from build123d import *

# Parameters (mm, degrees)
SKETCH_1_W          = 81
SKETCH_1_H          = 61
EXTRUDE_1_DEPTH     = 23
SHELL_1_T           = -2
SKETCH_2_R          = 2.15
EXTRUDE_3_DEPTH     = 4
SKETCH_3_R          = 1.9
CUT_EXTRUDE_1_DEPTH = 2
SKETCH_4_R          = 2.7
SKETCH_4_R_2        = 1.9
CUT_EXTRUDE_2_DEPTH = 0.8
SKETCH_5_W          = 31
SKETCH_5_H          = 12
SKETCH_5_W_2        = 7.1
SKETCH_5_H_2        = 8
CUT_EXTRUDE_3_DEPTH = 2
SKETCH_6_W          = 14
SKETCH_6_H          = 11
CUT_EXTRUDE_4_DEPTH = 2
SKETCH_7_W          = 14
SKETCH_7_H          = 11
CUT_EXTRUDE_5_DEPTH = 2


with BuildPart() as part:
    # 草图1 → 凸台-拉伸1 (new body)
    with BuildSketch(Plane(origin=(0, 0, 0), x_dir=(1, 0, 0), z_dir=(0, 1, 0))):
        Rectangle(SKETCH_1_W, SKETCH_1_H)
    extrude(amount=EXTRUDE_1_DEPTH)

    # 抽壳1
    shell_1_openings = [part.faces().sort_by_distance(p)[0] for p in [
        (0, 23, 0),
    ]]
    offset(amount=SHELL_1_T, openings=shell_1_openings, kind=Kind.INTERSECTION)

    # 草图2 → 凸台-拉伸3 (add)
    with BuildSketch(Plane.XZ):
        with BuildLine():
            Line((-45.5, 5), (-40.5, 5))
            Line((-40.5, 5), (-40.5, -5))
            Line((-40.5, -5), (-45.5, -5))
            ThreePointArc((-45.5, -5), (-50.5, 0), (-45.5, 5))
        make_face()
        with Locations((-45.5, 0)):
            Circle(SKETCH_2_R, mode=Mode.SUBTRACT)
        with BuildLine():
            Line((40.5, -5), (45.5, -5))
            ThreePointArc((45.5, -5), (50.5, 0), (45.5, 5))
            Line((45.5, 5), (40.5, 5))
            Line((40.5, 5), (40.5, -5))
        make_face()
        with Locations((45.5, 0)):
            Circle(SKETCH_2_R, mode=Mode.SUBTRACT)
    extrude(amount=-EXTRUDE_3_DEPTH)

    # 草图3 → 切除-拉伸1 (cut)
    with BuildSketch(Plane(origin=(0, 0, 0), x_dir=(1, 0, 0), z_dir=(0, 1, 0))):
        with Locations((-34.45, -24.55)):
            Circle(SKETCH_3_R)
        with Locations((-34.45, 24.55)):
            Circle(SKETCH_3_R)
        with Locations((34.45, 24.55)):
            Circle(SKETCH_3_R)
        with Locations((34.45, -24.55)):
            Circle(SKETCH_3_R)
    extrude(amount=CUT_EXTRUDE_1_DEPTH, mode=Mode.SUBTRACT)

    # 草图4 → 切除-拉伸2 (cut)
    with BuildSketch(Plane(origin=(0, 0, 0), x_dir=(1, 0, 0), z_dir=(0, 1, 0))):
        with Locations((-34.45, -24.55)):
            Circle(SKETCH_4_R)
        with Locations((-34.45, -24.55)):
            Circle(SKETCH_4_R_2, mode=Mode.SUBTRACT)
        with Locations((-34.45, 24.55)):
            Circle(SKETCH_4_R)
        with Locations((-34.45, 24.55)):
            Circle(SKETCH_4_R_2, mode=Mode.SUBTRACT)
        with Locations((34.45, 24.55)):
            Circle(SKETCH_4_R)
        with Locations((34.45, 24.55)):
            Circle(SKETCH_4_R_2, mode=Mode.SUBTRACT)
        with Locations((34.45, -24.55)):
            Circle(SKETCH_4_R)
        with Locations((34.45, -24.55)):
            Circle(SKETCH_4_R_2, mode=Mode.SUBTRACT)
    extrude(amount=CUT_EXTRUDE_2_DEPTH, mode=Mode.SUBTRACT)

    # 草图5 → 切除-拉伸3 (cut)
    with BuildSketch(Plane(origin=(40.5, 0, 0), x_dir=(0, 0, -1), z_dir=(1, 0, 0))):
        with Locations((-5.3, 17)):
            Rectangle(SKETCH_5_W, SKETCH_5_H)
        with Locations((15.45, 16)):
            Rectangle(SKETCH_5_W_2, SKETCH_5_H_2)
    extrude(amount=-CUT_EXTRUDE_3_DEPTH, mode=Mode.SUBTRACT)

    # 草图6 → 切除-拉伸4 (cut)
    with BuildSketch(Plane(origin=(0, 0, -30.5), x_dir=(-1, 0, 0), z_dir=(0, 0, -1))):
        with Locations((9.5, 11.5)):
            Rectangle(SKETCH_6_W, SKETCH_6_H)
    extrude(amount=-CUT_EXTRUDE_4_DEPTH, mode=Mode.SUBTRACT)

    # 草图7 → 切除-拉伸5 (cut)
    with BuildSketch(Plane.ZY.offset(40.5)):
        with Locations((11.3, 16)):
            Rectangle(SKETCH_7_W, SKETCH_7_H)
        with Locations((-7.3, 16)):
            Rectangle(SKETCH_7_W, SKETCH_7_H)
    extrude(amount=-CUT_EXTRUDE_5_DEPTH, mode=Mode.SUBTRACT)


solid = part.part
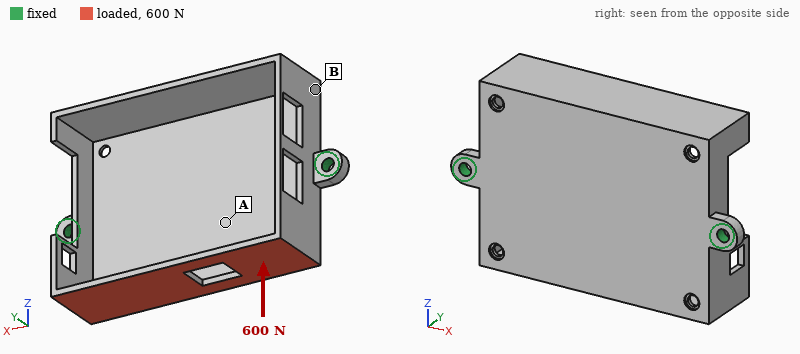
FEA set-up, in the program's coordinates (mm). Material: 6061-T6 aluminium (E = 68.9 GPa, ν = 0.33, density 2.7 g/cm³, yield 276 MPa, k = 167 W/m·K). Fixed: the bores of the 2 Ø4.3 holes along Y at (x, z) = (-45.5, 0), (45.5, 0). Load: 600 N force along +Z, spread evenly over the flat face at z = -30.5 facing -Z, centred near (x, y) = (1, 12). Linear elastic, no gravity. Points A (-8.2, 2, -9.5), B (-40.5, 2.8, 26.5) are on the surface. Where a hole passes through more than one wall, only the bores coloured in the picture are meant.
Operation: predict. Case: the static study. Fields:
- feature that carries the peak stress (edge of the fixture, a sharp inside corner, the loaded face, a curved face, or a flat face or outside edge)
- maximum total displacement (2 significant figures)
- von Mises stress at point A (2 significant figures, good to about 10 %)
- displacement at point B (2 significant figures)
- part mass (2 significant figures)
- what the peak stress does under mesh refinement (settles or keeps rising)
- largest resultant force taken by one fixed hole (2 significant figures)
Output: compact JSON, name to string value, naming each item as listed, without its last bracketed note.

{"feature that carries the peak stress": "edge of the fixture", "maximum total displacement": "0.41 mm", "von Mises stress at point A": "17 MPa", "displacement at point B": "0.079 mm", "part mass": "54 g", "what the peak stress does under mesh refinement": "keeps rising", "largest resultant force taken by one fixed hole": "310 N"}
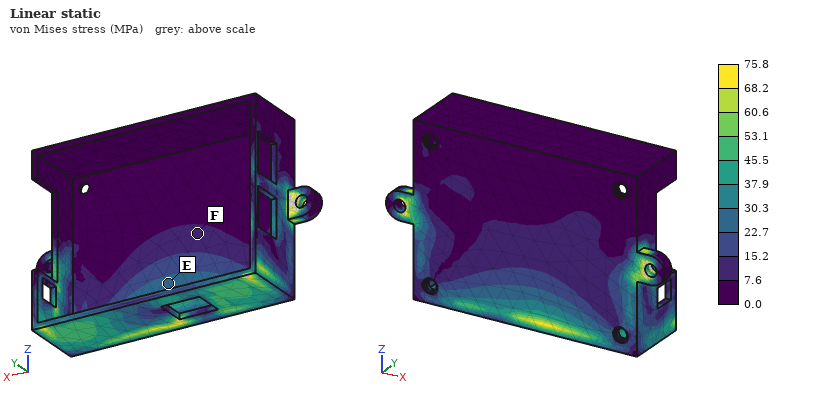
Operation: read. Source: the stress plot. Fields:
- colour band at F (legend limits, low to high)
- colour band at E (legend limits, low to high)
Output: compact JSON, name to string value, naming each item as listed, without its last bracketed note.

{"colour band at F": "7.6 to 15.2 MPa", "colour band at E": "22.7 to 30.3 MPa"}
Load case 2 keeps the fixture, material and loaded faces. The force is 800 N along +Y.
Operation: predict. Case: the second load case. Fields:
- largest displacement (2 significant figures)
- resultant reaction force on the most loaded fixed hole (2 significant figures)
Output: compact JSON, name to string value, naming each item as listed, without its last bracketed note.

{"largest displacement": "0.67 mm", "resultant reaction force on the most loaded fixed hole": "430 N"}
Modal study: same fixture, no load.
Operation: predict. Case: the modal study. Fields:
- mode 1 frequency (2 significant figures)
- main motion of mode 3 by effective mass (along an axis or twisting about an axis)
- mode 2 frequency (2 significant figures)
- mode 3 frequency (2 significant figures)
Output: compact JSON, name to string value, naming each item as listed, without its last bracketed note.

{"mode 1 frequency": "1200 Hz", "main motion of mode 3 by effective mass": "along Y", "mode 2 frequency": "1900 Hz", "mode 3 frequency": "2400 Hz"}
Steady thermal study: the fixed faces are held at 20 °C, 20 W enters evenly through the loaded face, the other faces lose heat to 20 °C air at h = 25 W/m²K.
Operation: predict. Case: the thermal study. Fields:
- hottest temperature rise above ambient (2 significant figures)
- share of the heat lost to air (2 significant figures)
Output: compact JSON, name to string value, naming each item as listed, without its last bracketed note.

{"hottest temperature rise above ambient": "32 K", "share of the heat lost to air": "31 %"}
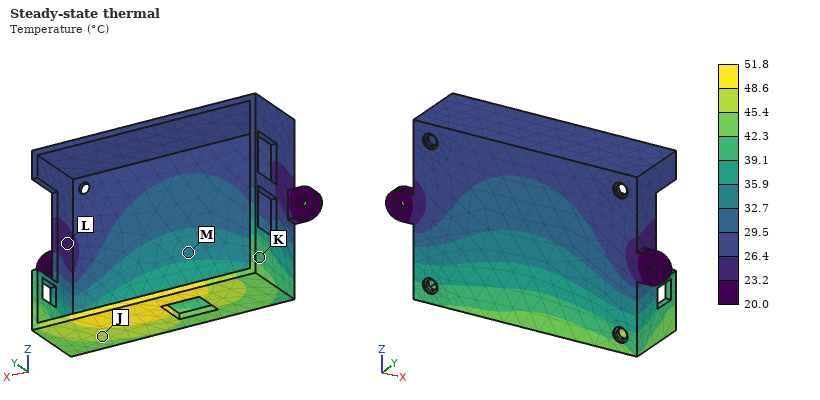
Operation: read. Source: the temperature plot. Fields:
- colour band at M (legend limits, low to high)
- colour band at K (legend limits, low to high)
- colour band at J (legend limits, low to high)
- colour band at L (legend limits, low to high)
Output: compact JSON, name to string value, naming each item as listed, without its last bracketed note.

{"colour band at M": "32.7 to 35.9 °C", "colour band at K": "39.1 to 42.3 °C", "colour band at J": "45.4 to 48.6 °C", "colour band at L": "23.2 to 26.4 °C"}
